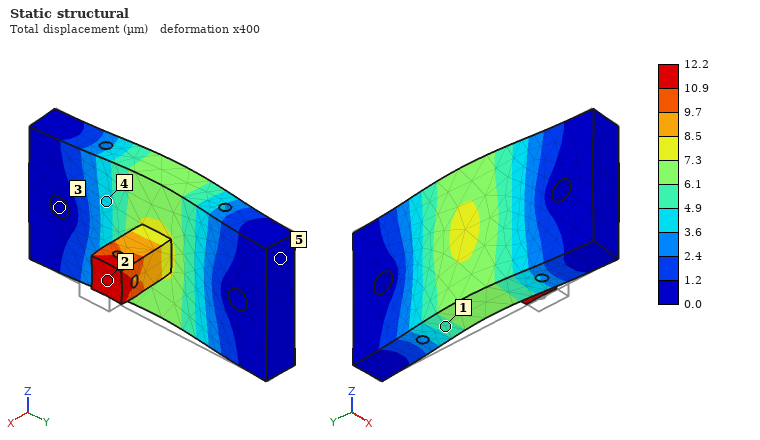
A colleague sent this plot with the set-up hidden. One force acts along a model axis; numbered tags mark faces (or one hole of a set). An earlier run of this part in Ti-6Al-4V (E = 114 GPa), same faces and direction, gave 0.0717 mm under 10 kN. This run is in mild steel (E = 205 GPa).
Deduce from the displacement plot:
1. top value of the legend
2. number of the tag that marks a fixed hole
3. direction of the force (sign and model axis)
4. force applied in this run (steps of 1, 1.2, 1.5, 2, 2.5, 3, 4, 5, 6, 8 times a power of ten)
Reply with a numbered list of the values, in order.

1. 12.2 µm
2. 3
3. -X
4. 3 kN
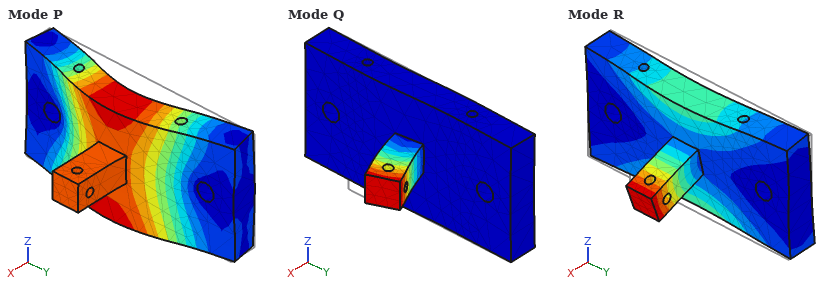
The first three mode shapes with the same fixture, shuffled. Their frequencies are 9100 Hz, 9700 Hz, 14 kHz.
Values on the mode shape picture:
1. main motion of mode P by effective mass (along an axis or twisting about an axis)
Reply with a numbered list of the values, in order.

1. along X
